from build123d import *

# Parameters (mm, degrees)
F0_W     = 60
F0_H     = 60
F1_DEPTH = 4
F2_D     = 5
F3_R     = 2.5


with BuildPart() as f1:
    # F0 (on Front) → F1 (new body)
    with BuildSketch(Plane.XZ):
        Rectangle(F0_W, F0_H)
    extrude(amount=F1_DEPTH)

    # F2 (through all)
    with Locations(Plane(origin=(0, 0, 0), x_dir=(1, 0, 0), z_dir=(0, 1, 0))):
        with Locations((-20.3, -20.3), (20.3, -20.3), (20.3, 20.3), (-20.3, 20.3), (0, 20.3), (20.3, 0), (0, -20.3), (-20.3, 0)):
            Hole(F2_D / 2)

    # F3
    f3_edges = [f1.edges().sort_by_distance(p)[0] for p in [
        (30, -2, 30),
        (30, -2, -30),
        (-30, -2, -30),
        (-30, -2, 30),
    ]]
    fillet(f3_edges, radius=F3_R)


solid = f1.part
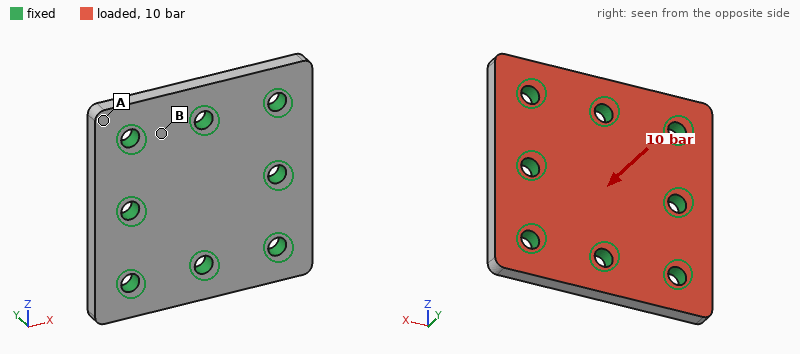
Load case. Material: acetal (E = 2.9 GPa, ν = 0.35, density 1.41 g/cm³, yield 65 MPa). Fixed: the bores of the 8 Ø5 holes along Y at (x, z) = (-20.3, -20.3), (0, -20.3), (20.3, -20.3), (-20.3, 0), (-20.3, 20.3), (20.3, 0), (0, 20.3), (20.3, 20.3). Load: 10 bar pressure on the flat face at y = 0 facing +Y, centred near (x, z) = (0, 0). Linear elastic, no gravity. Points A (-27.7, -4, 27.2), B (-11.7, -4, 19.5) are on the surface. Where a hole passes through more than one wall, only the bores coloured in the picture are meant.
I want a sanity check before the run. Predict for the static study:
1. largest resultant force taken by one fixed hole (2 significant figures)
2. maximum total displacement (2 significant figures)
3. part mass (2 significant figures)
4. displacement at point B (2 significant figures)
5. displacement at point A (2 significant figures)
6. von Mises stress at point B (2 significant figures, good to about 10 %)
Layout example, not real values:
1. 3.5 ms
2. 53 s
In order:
1. 490 N
2. 0.20 mm
3. 19 g
4. 0.033 mm
5. 0.059 mm
6. 7.7 MPa
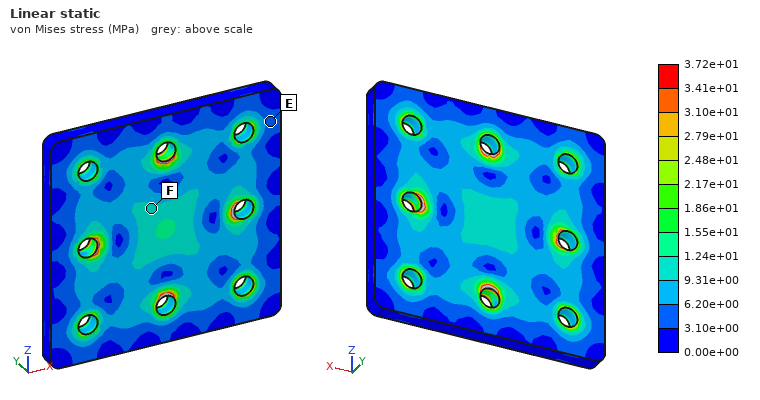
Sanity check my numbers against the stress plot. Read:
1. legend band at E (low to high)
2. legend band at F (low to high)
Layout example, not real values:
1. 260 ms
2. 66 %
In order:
1. 3.10e+00 to 6.20e+00 MPa
2. 9.31e+00 to 1.24e+01 MPa
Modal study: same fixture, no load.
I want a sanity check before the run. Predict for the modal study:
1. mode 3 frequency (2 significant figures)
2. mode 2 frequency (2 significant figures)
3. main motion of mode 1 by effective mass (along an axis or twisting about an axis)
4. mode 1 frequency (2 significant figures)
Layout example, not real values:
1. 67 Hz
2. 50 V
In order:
1. 9400 Hz
2. 9300 Hz
3. along Y
4. 5700 Hz
